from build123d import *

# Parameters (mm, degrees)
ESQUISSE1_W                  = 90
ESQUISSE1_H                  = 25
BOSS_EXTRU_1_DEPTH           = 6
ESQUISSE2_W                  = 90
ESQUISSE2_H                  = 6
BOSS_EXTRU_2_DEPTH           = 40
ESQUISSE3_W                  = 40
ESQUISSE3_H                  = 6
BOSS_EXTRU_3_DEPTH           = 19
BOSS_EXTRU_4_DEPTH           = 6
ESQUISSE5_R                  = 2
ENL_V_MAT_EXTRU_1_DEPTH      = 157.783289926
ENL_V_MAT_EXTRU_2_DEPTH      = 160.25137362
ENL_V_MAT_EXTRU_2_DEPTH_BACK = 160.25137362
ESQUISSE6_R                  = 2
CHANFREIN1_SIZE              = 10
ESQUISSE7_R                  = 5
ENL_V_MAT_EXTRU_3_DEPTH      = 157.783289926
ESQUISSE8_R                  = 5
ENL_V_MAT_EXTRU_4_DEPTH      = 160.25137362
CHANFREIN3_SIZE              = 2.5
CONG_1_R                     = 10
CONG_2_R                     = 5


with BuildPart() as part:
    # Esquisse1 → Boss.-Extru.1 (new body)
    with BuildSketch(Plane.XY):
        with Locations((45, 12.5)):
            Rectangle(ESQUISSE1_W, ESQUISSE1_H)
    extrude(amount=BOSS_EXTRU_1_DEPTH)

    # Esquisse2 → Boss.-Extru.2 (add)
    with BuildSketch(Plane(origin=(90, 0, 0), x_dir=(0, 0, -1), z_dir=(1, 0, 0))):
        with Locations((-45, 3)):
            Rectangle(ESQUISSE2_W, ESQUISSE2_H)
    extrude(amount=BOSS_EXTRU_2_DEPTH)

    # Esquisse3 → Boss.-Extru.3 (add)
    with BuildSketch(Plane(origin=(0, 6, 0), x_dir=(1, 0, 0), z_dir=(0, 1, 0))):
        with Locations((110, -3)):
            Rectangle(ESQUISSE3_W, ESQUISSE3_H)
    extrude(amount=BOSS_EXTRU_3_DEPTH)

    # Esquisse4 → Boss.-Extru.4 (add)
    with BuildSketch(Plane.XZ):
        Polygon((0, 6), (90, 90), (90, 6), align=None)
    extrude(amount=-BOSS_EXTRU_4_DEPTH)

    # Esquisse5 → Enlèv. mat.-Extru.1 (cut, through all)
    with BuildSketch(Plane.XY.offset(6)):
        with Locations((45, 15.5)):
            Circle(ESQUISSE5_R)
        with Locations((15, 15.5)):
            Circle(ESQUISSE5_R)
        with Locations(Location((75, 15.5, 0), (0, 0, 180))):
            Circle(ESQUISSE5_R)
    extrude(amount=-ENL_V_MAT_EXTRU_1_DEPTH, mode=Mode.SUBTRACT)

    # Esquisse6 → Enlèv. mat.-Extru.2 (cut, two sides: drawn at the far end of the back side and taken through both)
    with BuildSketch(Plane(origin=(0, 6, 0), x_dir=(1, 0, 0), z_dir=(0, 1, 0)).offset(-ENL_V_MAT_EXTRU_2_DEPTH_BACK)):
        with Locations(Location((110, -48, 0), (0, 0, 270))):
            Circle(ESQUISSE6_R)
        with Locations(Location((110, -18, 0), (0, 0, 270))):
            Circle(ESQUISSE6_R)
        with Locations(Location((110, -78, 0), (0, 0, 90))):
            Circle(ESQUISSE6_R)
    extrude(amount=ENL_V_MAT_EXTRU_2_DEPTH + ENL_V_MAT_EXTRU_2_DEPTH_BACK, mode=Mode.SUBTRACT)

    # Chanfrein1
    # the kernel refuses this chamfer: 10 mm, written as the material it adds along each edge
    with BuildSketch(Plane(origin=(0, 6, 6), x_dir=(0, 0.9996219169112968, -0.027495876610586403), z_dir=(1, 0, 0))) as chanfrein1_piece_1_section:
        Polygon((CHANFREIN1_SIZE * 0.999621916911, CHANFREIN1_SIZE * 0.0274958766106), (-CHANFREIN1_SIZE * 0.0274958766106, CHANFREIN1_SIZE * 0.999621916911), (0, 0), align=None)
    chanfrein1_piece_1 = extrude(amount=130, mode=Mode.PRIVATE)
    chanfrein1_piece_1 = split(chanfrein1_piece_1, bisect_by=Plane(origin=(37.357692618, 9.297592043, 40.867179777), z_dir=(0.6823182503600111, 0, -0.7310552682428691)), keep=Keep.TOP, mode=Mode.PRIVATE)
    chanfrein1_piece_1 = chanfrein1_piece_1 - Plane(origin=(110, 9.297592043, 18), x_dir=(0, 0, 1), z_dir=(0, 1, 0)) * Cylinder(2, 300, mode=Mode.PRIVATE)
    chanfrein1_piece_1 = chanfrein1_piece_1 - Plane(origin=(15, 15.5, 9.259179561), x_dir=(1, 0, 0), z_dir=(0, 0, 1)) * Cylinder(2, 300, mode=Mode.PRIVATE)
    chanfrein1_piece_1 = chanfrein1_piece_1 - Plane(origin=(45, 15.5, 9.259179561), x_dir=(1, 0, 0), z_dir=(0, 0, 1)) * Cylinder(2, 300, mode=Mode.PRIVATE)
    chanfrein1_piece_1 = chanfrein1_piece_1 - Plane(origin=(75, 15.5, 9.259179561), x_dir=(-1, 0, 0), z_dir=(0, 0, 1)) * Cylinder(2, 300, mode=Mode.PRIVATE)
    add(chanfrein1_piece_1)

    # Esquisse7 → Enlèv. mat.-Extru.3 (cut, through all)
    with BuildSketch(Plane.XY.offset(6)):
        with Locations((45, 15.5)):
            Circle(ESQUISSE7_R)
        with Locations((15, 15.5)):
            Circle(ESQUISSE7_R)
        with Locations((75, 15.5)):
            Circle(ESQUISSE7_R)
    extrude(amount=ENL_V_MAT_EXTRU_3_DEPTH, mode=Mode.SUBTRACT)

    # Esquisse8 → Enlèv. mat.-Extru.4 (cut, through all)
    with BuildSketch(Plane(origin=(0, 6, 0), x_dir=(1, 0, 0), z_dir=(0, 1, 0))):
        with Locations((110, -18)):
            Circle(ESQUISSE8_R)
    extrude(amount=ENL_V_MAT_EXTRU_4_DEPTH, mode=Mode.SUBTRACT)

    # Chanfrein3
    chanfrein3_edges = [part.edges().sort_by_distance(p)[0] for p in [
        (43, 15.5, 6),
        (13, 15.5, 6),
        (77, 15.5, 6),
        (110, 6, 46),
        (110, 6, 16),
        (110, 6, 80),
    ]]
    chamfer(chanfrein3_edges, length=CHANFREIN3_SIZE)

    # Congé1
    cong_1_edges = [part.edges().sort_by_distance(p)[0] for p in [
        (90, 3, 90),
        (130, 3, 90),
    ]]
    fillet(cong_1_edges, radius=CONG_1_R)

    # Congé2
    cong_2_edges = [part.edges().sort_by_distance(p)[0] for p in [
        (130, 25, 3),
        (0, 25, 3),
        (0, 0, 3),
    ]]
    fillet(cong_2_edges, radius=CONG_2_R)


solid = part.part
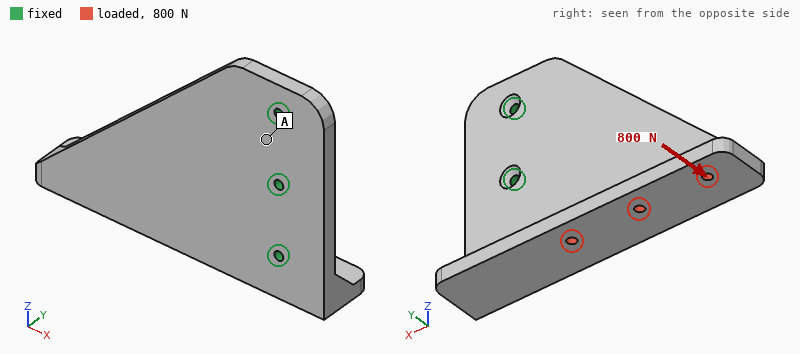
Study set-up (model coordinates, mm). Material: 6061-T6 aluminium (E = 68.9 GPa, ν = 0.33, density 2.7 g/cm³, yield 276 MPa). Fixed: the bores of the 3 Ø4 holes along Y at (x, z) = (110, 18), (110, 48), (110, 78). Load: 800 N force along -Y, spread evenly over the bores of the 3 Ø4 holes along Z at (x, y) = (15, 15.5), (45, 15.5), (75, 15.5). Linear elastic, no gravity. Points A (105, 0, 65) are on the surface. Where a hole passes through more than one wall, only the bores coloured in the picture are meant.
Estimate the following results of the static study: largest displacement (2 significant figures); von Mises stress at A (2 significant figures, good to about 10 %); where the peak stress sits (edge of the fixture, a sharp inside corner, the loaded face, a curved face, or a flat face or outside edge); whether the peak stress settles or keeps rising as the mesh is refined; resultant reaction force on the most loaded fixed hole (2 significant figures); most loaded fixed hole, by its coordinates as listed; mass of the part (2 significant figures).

1.4 mm
33 MPa
edge of the fixture
keeps rising
1.1 kN
(110, 18)
180 g
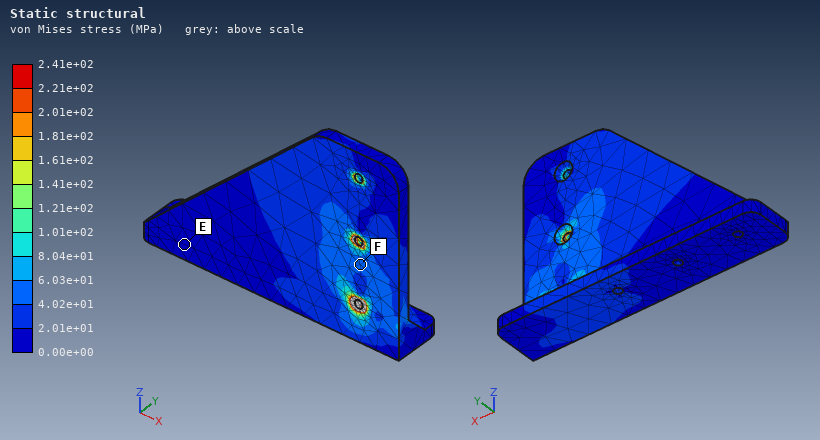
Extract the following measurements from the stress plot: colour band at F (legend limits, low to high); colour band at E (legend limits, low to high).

4.02e+01 to 6.03e+01 MPa
0.00e+00 to 2.01e+01 MPa
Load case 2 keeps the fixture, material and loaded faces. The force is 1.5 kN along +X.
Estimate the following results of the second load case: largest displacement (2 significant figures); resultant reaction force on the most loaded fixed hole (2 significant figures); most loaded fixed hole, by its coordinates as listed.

0.49 mm
1.8 kN
(110, 18)
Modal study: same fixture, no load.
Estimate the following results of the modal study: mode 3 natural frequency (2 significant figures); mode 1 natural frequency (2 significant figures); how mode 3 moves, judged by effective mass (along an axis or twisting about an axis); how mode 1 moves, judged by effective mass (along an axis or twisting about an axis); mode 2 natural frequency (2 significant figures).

3700 Hz
550 Hz
along Z
along Y
2100 Hz
